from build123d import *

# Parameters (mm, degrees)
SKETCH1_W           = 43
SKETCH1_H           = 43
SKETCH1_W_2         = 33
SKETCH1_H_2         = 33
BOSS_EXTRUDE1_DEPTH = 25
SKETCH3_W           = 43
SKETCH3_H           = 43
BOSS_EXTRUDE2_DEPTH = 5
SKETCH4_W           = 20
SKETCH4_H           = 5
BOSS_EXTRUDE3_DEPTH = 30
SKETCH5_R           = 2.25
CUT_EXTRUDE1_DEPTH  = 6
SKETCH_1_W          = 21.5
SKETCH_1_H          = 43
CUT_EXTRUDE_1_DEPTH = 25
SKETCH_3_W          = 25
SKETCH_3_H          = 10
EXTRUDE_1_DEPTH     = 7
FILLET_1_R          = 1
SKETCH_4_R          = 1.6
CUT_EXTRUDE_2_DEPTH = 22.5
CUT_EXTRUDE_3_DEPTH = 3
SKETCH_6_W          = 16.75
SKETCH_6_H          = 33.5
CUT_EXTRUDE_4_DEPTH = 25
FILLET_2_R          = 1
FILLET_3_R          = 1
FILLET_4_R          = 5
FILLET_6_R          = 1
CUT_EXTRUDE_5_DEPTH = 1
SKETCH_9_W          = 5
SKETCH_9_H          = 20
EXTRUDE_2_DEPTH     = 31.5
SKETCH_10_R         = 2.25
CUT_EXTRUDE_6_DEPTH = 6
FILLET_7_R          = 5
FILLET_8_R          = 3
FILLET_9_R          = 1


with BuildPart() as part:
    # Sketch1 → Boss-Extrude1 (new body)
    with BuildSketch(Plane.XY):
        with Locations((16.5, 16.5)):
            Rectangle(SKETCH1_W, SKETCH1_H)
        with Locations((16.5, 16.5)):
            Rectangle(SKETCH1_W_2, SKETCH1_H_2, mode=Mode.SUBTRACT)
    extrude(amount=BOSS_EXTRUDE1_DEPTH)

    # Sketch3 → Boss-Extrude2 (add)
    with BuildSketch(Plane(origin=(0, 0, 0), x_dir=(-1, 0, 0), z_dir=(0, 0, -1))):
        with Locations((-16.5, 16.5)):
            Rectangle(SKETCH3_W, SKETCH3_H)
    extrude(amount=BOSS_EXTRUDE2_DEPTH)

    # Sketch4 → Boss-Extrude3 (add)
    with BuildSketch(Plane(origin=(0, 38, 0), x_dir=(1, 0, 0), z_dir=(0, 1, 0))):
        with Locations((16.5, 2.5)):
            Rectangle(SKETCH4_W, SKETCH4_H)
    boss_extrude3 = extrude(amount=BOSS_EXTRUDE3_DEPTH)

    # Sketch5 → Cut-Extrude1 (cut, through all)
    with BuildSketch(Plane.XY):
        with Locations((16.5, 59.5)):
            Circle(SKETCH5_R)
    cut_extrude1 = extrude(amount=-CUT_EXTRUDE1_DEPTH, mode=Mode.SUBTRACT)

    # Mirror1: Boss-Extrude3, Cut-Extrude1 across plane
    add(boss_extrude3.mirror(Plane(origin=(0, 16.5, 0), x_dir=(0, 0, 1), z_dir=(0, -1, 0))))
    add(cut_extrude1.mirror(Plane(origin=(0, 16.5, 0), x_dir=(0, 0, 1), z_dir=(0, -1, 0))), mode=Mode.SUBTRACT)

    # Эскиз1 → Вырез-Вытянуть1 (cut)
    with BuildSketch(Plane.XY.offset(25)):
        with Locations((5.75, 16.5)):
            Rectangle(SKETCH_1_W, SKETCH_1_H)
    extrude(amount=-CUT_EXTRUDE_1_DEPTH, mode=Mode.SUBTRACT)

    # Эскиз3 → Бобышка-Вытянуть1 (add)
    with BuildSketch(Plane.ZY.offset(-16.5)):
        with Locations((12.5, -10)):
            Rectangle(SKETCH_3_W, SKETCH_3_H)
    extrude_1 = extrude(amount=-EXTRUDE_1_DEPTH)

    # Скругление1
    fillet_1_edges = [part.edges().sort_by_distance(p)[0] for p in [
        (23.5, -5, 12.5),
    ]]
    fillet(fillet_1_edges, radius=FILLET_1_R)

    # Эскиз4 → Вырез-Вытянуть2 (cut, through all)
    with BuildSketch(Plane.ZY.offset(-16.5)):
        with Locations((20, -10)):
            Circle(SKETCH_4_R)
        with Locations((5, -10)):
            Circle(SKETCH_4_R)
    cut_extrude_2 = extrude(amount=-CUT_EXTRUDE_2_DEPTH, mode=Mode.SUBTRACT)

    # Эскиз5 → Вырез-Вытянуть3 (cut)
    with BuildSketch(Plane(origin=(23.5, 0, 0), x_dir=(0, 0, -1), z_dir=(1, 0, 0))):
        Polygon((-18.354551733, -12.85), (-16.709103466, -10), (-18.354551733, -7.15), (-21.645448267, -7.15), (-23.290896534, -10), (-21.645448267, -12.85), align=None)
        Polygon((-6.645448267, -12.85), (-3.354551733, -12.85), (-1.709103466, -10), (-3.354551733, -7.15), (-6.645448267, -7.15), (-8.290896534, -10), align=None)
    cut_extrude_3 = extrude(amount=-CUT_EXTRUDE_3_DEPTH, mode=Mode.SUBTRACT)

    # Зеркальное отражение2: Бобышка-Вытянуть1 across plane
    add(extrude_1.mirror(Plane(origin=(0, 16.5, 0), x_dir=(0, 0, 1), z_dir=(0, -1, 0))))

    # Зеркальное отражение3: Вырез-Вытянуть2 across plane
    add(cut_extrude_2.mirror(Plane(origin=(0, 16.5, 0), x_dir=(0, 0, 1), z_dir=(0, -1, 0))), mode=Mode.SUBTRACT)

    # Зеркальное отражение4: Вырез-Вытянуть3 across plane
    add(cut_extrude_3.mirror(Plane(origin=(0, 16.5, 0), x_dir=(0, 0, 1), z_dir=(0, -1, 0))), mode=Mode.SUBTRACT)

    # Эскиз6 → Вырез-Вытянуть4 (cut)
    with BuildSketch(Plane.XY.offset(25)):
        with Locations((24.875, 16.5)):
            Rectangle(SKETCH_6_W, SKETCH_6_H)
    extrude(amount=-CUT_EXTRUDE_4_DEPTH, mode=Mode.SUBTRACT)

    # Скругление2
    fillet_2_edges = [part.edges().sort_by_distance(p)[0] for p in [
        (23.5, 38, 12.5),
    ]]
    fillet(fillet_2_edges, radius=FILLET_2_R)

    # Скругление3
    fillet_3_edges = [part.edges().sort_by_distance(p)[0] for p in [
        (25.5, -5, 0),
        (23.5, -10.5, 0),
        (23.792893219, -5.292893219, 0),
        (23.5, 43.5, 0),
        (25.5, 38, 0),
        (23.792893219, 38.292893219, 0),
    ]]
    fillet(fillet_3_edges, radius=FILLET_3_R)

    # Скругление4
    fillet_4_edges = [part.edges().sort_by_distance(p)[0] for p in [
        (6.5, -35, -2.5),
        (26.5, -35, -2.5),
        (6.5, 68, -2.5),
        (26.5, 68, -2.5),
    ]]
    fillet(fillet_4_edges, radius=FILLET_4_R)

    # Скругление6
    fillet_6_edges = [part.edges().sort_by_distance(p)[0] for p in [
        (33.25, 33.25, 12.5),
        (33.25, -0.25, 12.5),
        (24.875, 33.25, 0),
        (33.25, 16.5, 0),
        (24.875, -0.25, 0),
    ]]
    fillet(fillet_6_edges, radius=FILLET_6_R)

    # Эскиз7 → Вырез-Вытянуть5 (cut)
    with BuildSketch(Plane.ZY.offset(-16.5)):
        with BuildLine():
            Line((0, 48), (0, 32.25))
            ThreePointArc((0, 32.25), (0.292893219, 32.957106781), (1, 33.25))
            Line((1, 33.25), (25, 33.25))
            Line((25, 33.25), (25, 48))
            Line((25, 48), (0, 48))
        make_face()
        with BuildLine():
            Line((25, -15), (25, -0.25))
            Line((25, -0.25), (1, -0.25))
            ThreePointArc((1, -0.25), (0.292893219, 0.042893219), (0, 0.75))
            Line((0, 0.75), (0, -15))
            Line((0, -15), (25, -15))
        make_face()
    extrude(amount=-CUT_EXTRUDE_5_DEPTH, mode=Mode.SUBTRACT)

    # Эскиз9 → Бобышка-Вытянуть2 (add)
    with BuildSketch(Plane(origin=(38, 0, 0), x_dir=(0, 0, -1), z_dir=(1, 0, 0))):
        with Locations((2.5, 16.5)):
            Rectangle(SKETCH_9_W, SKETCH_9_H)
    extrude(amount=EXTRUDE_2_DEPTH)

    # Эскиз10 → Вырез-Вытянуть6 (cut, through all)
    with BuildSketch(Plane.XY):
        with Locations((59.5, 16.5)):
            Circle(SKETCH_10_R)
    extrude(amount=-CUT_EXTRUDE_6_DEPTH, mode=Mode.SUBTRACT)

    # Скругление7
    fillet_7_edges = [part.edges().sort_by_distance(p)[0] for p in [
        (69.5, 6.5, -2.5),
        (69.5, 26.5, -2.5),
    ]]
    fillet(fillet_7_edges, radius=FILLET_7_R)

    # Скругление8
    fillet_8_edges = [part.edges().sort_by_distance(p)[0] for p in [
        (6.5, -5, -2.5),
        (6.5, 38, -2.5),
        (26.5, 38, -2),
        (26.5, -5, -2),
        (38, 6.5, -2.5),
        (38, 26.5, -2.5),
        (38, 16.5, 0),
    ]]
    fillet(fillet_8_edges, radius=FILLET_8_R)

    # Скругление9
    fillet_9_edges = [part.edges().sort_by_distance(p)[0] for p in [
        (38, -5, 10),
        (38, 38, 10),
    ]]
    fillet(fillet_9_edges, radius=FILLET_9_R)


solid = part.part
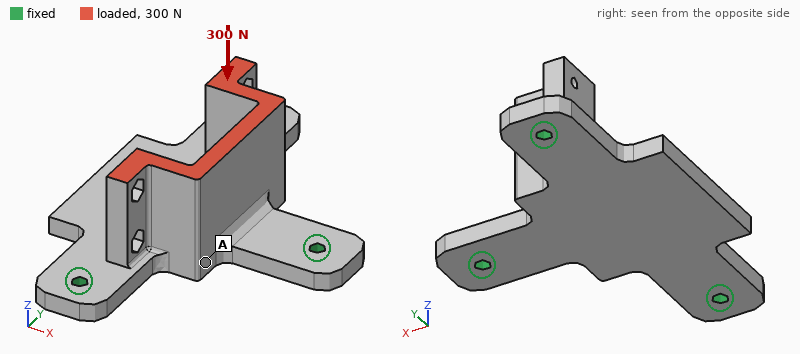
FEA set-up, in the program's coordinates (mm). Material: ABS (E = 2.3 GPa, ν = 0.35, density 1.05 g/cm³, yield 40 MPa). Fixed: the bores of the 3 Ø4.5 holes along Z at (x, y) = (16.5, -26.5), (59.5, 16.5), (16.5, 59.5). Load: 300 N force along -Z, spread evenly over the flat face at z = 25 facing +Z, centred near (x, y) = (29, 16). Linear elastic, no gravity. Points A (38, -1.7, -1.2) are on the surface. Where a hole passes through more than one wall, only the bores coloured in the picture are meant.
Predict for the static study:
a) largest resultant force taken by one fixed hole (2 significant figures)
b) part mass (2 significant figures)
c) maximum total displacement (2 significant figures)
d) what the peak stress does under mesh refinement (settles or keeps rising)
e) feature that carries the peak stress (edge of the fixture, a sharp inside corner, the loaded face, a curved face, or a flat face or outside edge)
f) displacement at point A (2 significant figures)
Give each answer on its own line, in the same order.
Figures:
110 N
31 g
0.25 mm
keeps rising
edge of the fixture
0.22 mm
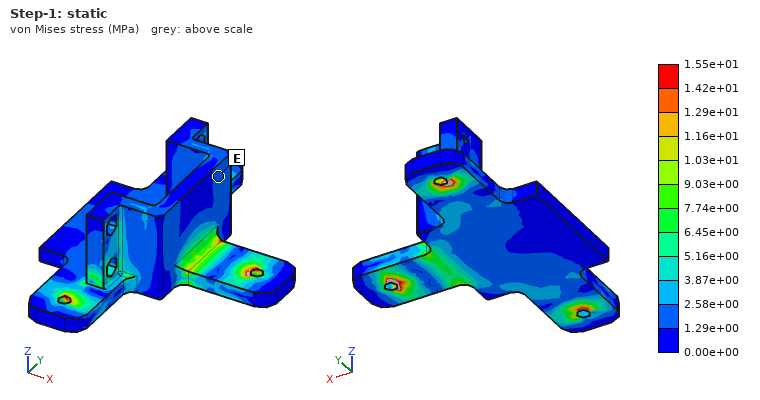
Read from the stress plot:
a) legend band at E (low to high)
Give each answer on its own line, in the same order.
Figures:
1.29e+00 to 2.58e+00 MPa
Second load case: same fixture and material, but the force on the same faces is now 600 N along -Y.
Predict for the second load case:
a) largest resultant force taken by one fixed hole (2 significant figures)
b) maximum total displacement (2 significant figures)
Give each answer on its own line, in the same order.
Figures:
350 N
0.80 mm
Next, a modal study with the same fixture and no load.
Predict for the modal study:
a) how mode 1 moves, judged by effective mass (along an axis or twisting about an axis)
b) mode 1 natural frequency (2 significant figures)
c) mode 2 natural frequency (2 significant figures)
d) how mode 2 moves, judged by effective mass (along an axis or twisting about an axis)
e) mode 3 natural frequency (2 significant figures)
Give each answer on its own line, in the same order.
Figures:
along Z
960 Hz
1300 Hz
along Z
1700 Hz
